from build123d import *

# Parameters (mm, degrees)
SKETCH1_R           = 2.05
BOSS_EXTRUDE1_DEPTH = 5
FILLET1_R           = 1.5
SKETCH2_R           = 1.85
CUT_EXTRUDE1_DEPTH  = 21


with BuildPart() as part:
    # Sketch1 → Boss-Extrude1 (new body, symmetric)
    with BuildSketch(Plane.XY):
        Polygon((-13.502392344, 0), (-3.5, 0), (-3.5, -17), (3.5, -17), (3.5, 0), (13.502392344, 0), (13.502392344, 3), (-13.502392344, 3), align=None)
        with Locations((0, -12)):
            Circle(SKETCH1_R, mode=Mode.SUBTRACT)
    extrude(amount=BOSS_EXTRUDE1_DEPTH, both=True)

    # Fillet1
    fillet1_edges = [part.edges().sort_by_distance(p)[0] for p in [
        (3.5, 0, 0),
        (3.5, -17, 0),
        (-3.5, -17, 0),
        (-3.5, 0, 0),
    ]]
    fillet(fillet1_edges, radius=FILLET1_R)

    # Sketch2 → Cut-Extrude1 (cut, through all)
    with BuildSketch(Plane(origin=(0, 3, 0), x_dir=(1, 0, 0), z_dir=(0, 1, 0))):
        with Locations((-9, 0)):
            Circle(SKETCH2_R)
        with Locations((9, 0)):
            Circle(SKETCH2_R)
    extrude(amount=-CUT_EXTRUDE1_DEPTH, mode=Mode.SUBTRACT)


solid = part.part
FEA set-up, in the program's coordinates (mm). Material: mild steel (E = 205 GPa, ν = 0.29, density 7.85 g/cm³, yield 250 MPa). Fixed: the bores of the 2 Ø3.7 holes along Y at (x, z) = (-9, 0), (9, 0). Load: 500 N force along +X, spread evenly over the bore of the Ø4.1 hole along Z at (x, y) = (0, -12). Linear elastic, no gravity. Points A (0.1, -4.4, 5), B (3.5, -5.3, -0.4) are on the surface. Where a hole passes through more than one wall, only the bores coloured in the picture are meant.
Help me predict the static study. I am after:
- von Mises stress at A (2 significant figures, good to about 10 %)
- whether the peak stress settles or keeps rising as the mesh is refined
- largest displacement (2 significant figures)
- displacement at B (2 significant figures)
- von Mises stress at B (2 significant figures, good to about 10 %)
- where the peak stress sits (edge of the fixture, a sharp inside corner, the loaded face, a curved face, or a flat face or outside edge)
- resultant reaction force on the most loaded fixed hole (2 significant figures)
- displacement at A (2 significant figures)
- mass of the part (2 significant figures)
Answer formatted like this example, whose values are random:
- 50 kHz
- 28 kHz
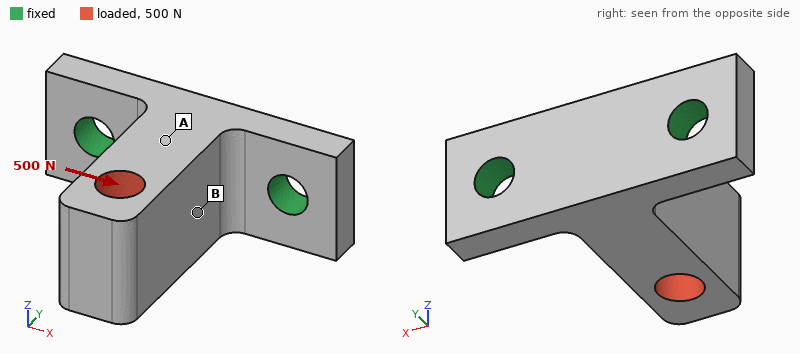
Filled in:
- 21 MPa
- keeps rising
- 19 µm
- 5.8 µm
- 42 MPa
- edge of the fixture
- 590 N
- 3.7 µm
- 14 g
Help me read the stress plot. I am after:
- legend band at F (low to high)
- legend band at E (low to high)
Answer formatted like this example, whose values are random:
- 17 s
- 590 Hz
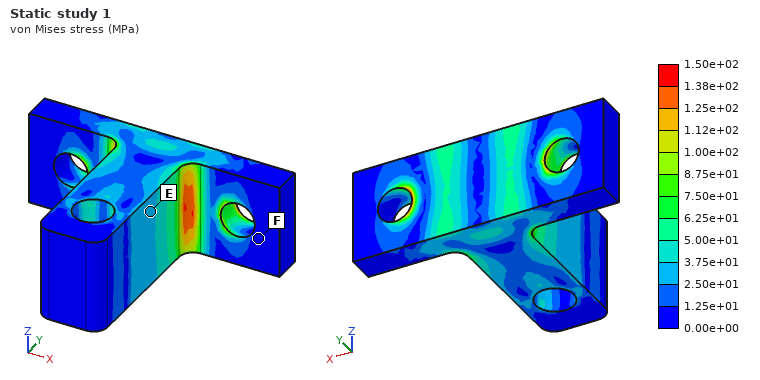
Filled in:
- 0.00e+00 to 1.25e+01 MPa
- 2.50e+01 to 3.75e+01 MPa
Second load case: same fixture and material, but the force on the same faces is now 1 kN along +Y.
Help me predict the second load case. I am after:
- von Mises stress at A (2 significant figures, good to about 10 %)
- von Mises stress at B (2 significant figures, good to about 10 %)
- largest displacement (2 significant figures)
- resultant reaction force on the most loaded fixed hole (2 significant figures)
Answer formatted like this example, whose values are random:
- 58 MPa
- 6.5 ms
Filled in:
- 11 MPa
- 16 MPa
- 4.1 µm
- 540 N
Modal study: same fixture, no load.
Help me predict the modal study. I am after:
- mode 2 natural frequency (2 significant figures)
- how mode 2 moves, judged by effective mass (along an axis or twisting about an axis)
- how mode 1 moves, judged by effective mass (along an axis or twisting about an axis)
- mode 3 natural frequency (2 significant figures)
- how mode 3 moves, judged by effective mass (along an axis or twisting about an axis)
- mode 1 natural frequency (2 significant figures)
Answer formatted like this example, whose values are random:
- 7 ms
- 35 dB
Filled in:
- 14 kHz
- along X
- along Z
- 28 kHz
- along Y
- 8500 Hz
